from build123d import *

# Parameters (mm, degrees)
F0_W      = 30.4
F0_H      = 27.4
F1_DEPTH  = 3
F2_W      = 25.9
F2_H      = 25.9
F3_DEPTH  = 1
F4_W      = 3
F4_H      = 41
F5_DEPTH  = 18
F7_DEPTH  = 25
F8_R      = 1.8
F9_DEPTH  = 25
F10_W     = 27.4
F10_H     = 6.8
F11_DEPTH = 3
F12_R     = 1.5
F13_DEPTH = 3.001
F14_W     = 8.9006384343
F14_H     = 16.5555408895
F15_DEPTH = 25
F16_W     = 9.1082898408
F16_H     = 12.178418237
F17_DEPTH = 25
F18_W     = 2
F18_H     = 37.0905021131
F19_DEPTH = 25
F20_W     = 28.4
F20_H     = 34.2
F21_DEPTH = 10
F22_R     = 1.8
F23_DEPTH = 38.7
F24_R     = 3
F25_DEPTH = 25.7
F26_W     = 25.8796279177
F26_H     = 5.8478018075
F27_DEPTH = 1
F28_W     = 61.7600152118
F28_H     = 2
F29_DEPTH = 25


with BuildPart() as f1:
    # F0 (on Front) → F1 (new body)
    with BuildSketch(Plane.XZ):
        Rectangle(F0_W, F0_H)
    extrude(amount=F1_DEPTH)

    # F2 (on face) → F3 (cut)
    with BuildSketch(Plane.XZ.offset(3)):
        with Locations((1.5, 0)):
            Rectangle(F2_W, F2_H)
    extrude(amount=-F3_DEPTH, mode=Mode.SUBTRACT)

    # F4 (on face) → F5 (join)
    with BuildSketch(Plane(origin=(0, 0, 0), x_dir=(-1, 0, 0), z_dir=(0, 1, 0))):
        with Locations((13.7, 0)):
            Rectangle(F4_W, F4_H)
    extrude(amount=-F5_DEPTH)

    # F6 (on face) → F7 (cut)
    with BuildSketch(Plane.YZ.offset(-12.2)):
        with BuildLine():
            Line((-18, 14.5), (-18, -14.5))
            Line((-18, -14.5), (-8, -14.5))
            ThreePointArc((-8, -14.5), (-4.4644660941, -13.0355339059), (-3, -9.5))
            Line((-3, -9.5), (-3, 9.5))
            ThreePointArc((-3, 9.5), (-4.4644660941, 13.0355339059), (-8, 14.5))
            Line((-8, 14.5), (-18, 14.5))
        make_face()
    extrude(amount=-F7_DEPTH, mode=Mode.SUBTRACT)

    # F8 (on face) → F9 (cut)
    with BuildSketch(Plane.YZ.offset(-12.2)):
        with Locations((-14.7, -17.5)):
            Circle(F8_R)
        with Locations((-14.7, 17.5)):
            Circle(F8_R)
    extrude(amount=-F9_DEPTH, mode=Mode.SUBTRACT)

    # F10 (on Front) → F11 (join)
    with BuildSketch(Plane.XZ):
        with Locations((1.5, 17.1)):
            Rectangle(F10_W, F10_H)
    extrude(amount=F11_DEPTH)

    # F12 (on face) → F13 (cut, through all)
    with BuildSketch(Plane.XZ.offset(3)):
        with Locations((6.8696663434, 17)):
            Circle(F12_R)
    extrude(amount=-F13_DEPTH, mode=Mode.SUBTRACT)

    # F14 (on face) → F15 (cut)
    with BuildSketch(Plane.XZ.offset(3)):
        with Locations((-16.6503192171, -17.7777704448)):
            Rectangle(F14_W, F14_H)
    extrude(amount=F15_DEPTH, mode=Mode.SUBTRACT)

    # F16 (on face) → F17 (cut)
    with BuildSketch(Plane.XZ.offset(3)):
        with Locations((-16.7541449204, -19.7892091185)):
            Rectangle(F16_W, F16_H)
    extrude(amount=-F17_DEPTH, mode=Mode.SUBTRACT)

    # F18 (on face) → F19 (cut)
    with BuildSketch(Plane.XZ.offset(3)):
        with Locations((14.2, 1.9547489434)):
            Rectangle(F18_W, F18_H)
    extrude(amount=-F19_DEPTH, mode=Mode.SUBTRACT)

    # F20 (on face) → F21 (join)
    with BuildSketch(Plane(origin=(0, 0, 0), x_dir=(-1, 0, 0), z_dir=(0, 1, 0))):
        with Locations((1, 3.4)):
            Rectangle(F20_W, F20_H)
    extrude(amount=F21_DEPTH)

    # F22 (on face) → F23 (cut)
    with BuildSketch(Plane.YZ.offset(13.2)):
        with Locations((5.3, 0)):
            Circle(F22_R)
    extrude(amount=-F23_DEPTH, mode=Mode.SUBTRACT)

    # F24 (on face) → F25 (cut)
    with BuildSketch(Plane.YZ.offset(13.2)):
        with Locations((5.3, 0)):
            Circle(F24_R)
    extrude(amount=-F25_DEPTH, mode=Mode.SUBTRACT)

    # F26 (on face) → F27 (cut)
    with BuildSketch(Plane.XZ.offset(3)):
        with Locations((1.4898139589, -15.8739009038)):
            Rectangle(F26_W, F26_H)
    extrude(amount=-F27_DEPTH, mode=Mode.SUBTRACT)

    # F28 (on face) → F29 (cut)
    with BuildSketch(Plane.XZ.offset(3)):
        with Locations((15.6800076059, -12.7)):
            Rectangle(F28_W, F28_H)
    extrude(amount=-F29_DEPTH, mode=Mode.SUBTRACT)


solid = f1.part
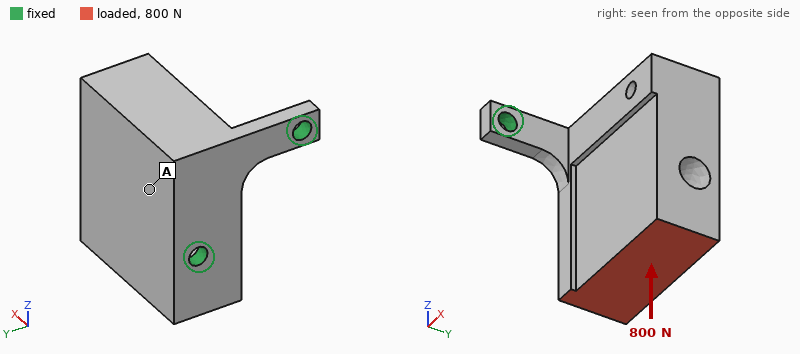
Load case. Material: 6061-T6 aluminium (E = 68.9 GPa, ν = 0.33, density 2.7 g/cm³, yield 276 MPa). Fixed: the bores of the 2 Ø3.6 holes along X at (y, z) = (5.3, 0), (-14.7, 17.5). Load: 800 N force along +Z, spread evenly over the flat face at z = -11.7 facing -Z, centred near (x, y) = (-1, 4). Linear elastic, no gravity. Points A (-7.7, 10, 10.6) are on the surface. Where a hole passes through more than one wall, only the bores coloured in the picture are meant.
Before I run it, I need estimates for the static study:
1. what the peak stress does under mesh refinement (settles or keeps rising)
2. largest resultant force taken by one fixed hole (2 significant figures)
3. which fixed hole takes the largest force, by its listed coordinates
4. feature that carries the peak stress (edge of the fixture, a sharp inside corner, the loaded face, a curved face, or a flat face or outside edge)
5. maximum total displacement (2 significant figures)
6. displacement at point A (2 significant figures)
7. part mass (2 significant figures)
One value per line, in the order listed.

keeps rising
790 N
(5.3, 0)
edge of the fixture
0.12 mm
0.046 mm
29 g
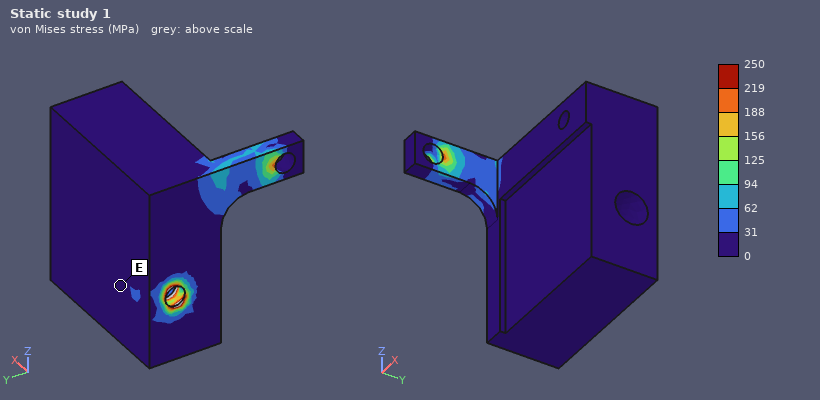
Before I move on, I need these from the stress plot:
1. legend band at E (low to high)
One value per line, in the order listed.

0 to 31 MPa
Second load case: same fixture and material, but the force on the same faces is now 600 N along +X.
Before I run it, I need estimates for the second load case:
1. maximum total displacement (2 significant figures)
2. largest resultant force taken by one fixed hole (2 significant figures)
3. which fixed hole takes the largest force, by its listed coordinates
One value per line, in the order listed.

88 µm
730 N
(5.3, 0)
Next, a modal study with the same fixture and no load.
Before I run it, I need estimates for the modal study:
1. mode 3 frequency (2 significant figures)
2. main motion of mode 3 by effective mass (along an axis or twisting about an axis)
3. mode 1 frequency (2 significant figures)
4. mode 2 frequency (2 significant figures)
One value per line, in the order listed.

11 kHz
twisting about X
2500 Hz
3700 Hz
